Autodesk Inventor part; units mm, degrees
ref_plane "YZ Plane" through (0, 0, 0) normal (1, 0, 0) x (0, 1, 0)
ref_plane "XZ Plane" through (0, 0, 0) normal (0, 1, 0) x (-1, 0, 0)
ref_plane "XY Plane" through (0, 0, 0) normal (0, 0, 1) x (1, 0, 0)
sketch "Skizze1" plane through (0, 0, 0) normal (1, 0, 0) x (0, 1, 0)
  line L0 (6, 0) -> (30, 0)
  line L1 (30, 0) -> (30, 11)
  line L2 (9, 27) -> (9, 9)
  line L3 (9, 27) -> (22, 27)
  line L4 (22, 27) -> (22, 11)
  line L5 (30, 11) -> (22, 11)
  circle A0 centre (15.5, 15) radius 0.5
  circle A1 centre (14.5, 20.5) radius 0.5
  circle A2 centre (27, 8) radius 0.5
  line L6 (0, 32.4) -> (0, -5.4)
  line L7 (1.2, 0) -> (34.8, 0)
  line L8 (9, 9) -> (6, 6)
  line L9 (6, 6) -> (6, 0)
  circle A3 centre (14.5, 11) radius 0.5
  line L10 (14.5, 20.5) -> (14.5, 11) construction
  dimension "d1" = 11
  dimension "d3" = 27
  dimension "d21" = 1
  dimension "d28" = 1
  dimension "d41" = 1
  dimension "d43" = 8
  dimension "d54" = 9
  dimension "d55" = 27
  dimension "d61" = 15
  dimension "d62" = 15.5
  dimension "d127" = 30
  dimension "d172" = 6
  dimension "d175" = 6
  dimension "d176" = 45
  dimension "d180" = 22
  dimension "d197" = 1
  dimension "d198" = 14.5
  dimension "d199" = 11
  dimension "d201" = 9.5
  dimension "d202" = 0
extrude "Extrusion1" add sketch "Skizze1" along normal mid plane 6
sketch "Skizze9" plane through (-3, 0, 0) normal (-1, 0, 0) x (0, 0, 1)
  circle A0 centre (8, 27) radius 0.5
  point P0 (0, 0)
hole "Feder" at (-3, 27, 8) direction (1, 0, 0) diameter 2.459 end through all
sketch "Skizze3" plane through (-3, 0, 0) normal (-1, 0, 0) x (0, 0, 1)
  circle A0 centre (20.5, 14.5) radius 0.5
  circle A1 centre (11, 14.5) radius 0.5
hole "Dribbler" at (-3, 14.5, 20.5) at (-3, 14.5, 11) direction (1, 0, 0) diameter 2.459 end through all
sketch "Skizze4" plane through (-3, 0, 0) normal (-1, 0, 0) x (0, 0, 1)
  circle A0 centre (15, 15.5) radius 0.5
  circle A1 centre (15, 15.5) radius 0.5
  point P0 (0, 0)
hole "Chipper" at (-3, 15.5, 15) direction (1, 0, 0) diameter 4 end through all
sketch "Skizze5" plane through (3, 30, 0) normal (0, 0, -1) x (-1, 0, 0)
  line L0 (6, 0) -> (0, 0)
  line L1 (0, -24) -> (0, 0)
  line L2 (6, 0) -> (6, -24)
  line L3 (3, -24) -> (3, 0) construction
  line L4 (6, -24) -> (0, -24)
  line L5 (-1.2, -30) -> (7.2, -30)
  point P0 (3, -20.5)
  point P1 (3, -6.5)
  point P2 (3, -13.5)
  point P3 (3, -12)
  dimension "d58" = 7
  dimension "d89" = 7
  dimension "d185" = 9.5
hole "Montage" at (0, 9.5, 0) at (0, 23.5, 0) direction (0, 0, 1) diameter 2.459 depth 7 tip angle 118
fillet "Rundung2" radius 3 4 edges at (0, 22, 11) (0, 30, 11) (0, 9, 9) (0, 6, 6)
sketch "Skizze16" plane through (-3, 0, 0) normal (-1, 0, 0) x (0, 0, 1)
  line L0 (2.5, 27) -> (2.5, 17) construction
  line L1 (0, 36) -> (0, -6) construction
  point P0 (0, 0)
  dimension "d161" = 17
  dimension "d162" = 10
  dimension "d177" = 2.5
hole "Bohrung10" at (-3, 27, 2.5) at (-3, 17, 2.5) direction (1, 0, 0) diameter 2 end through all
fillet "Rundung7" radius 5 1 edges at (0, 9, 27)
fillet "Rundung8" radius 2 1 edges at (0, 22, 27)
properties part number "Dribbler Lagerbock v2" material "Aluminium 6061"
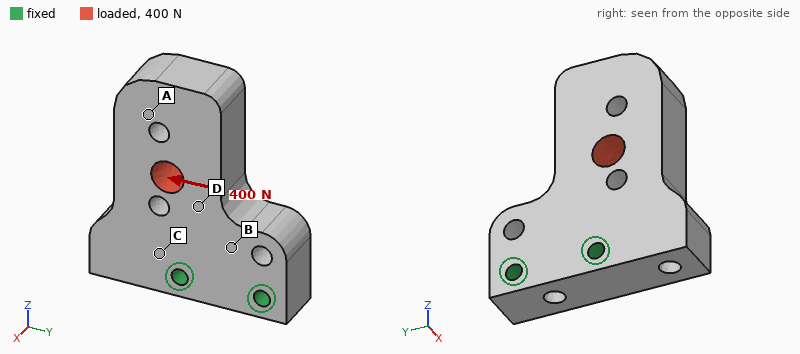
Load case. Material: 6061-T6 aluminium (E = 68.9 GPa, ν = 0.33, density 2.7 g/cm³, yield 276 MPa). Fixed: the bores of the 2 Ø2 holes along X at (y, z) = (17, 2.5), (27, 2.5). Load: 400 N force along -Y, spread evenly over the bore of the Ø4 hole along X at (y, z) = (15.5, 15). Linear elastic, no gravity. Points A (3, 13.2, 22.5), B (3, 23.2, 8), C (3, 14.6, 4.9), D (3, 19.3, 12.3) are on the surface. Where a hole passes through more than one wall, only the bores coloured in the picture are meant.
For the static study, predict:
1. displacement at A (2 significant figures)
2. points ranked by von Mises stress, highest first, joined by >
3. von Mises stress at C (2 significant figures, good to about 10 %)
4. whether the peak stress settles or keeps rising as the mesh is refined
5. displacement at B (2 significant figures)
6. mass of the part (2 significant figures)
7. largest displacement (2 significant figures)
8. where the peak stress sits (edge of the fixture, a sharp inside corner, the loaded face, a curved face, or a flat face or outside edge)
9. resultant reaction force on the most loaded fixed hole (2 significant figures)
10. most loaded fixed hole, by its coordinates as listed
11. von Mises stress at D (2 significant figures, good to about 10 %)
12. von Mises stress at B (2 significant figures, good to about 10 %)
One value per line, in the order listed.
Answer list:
11 µm
B > D > C > A
8.1 MPa
keeps rising
2.0 µm
6.7 g
13 µm
edge of the fixture
490 N
(27, 2.5)
14 MPa
20 MPa
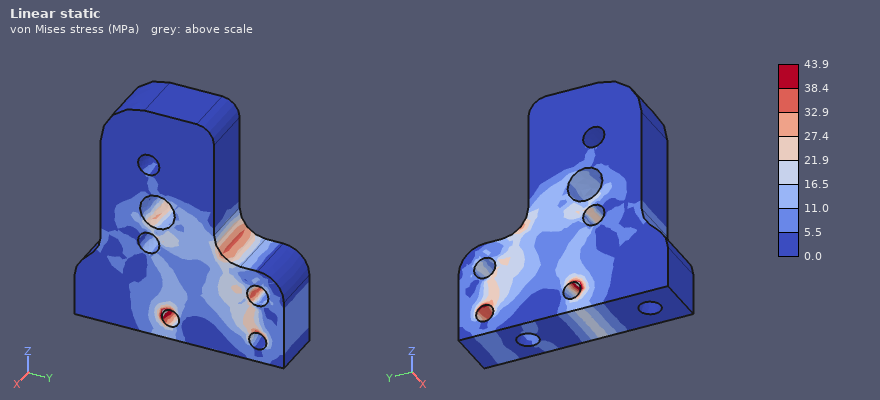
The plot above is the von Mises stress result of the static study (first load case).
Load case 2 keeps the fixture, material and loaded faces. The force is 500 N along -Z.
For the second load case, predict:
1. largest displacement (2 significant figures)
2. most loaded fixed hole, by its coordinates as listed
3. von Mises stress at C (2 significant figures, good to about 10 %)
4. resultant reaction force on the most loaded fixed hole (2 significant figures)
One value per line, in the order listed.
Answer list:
5.6 µm
(17, 2.5)
10 MPa
530 N
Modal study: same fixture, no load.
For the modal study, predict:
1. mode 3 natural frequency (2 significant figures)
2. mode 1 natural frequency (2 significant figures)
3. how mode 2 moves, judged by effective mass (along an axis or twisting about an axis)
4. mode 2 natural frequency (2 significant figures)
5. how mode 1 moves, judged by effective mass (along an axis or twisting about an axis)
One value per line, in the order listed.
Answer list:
22 kHz
7800 Hz
along Y
14 kHz
along X
